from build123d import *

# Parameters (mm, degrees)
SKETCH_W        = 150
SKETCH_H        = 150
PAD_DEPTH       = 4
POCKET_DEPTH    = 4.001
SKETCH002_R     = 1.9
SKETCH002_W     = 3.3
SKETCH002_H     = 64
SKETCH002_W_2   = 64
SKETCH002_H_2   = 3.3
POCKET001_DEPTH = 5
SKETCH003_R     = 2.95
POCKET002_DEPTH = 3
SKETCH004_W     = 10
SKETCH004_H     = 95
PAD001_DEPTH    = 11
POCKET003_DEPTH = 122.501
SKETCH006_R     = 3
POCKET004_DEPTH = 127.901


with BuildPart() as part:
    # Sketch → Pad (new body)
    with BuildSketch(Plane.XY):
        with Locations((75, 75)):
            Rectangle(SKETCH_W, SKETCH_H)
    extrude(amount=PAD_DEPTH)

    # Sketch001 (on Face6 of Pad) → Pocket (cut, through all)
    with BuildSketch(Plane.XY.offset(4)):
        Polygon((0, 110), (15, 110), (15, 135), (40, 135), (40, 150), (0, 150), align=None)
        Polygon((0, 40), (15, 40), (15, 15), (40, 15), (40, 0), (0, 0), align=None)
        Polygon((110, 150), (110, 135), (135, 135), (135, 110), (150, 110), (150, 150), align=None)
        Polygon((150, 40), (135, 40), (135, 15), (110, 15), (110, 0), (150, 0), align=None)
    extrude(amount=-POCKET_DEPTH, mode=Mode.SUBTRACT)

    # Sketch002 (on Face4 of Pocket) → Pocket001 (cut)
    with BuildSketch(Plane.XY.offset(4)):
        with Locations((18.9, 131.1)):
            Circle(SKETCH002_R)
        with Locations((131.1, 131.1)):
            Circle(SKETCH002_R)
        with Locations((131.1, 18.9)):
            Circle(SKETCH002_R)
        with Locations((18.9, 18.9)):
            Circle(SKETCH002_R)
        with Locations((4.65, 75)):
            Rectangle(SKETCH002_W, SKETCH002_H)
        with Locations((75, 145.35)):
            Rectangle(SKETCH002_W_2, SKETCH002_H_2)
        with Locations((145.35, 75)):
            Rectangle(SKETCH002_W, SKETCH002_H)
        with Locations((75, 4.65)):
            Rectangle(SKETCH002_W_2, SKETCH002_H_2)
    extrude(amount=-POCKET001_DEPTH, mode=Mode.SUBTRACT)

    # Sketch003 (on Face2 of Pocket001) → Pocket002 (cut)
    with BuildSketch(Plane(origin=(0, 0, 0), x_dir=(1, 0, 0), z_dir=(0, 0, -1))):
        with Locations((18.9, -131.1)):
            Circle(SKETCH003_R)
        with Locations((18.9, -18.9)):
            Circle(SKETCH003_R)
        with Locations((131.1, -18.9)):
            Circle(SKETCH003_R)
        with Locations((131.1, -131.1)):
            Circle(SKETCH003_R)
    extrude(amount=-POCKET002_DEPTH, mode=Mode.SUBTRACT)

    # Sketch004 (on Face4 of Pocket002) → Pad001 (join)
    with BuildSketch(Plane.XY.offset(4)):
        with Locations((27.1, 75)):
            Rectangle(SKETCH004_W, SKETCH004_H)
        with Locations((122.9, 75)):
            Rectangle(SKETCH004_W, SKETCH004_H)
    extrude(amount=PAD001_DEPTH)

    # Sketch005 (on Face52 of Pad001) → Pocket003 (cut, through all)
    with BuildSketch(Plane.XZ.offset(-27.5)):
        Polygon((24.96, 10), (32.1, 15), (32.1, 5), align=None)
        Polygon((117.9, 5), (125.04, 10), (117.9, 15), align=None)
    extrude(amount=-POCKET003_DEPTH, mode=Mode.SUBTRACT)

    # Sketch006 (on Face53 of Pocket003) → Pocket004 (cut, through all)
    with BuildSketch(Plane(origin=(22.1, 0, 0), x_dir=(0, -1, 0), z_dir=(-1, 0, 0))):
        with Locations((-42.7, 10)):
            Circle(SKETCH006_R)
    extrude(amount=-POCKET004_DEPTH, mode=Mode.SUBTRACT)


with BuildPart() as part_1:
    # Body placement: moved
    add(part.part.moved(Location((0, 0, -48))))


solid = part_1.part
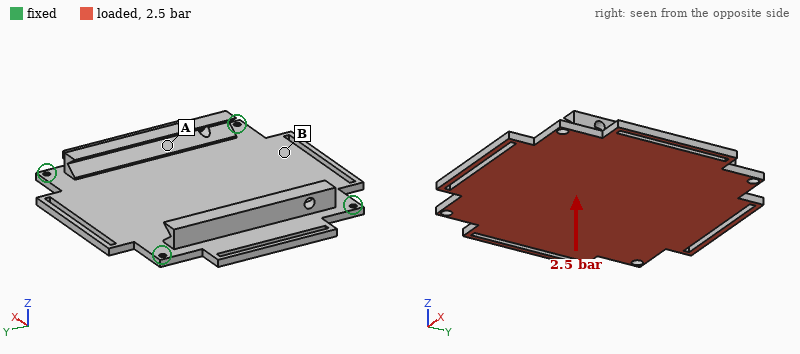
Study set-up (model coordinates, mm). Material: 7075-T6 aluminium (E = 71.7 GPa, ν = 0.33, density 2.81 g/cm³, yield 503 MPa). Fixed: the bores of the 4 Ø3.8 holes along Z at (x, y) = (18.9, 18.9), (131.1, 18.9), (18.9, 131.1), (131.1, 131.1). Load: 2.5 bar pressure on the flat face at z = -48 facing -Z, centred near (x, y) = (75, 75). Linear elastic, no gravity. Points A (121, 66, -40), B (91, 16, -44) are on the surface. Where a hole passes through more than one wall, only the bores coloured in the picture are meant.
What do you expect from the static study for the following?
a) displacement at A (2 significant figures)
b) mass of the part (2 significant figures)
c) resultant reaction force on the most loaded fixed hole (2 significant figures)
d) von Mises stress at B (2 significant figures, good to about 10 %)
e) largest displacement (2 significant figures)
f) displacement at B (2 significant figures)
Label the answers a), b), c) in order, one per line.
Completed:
a) 0.31 mm
b) 240 g
c) 2.6 kN
d) 71 MPa
e) 0.79 mm
f) 0.68 mm
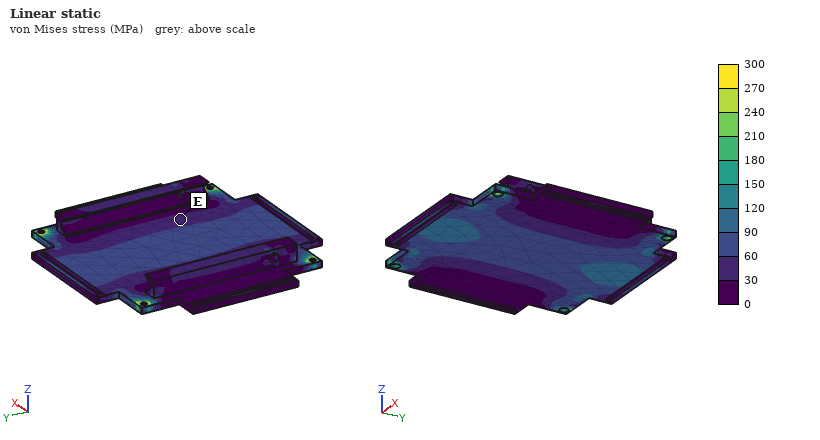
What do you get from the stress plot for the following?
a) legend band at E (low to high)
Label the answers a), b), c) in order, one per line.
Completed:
a) 30 to 60 MPa
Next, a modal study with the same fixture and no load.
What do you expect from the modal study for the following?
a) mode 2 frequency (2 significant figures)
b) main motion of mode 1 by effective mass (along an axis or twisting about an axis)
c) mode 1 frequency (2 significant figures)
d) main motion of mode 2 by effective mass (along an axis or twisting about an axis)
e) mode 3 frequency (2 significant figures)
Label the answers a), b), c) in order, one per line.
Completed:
a) 1400 Hz
b) along Z
c) 920 Hz
d) twisting about X
e) 1900 Hz
